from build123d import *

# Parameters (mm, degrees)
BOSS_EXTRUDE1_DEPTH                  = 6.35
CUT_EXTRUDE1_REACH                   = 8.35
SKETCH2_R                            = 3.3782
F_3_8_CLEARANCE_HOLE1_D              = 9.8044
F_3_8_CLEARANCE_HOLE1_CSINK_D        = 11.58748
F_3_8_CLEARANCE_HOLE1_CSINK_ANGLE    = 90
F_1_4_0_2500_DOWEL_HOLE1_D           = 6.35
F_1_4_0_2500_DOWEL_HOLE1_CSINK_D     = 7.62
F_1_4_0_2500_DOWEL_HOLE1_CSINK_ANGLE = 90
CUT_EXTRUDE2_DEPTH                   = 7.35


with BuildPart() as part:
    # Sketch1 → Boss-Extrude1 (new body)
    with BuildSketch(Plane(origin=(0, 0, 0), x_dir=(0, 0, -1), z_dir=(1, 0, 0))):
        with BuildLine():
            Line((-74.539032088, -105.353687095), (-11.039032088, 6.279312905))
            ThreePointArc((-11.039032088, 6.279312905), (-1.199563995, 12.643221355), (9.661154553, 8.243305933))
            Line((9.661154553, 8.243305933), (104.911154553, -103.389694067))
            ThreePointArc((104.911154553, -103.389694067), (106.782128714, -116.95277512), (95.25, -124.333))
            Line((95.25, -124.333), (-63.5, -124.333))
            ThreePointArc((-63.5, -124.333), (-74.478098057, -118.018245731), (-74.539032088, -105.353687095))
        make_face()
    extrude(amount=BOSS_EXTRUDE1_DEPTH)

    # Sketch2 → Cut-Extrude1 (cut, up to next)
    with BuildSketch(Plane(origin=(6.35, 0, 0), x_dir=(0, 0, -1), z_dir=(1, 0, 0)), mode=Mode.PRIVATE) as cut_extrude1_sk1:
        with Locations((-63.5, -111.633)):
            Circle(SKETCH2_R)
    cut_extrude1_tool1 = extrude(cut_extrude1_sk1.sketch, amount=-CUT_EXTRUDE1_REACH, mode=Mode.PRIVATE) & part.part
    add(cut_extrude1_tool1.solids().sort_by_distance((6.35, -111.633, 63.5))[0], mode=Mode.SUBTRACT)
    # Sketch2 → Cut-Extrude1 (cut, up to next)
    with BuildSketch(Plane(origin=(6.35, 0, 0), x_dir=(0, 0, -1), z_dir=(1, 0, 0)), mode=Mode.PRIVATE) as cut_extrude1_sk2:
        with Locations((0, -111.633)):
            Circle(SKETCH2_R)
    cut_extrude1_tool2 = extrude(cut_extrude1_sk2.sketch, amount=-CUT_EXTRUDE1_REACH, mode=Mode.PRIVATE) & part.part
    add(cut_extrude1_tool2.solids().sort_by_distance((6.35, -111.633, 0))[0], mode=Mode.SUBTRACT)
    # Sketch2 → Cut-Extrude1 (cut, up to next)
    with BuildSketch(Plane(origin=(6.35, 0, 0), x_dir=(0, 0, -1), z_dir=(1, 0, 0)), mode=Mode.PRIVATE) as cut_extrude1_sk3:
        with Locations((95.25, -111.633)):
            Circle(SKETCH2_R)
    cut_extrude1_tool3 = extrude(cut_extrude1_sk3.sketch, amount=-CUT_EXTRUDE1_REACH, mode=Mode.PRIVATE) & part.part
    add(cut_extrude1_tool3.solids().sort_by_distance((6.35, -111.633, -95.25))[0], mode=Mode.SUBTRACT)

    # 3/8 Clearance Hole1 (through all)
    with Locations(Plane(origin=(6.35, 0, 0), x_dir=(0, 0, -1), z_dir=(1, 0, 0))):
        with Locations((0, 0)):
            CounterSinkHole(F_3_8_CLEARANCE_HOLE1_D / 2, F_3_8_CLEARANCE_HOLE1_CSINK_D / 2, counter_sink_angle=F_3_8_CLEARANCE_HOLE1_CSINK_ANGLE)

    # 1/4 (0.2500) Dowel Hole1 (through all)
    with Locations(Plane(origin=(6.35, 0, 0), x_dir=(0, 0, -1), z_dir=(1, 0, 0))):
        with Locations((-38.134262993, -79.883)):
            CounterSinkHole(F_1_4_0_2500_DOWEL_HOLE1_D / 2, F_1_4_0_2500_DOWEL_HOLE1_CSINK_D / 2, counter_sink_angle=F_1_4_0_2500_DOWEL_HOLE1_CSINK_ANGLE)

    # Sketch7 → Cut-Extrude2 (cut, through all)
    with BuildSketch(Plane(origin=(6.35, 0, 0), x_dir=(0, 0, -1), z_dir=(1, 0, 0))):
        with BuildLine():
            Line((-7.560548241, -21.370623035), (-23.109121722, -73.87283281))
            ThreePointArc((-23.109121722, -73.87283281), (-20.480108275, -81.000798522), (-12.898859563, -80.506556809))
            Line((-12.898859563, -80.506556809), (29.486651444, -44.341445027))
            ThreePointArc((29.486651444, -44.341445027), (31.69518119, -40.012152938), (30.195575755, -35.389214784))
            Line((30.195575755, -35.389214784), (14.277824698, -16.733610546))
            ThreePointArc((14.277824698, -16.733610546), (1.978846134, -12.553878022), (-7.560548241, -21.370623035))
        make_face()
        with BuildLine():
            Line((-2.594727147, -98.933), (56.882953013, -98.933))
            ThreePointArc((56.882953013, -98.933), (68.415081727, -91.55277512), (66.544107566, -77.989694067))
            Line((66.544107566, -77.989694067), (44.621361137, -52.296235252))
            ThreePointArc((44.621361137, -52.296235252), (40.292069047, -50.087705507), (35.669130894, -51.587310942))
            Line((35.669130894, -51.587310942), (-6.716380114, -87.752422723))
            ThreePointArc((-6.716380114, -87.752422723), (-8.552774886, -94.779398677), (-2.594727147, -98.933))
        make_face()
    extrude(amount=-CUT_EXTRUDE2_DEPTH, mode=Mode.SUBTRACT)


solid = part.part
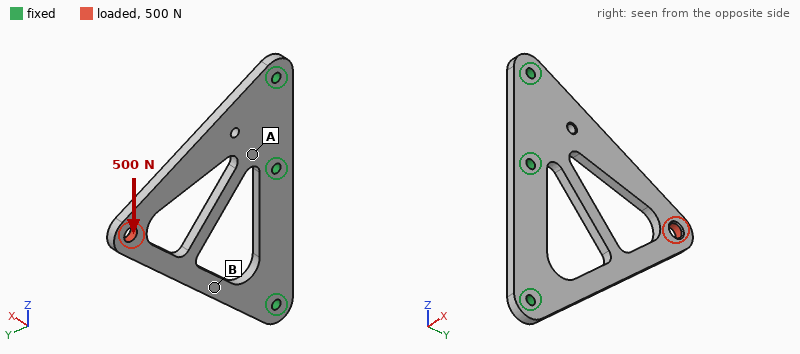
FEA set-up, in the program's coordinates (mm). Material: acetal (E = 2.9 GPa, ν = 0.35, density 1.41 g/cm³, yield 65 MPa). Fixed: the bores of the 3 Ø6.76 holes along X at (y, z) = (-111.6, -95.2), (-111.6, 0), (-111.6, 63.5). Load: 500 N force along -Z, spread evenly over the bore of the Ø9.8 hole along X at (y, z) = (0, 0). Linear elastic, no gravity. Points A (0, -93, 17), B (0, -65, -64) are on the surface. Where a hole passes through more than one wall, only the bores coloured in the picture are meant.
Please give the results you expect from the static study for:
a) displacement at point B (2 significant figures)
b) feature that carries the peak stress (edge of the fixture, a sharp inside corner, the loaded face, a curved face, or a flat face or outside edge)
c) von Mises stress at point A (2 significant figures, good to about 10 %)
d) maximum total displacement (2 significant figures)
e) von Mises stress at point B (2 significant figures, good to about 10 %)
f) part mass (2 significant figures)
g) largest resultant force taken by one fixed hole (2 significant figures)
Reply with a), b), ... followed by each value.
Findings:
a) 0.095 mm
b) the loaded face
c) 1.8 MPa
d) 0.38 mm
e) 4.9 MPa
f) 91 g
g) 410 N
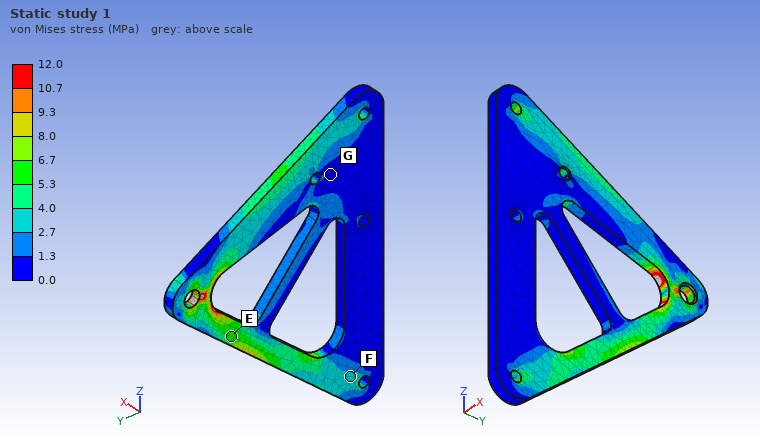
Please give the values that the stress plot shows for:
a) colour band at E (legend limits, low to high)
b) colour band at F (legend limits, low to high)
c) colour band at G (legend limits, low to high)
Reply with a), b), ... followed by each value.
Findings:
a) 5.3 to 6.7 MPa
b) 2.7 to 4.0 MPa
c) 0.0 to 1.3 MPa
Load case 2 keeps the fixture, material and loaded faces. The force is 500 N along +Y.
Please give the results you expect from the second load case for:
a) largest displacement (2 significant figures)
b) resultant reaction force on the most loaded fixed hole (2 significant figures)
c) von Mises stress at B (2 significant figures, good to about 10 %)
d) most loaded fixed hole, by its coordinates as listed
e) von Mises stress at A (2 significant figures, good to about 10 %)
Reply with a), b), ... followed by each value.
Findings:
a) 0.63 mm
b) 290 N
c) 3.3 MPa
d) (-111.6, 63.5)
e) 0.71 MPa
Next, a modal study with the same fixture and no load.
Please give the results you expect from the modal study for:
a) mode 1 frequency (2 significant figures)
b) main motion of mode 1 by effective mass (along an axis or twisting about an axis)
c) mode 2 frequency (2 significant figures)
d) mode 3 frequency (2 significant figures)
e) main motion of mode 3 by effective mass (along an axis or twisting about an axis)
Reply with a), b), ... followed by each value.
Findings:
a) 120 Hz
b) along X
c) 390 Hz
d) 570 Hz
e) along X
